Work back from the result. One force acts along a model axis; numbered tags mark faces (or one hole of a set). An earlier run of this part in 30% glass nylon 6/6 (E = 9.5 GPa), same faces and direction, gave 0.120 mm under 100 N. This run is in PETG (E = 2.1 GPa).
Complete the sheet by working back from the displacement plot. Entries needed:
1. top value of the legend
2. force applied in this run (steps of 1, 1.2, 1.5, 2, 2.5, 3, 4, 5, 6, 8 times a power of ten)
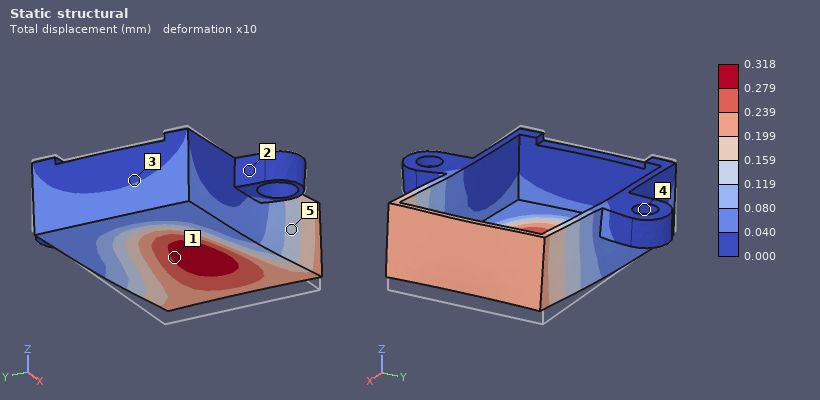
0.318 mm
60 N
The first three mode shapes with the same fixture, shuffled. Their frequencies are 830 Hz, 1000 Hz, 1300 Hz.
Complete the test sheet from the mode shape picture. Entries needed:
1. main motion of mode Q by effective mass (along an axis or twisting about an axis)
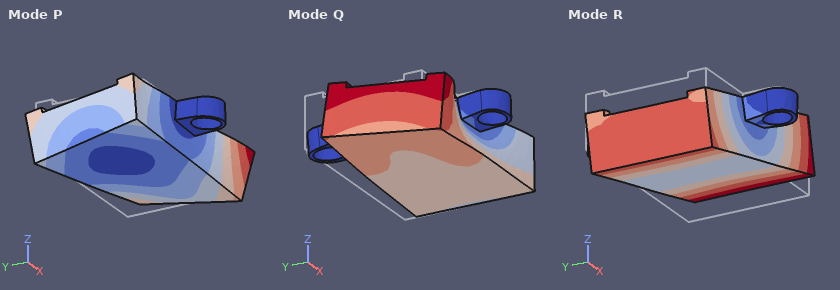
along Y
